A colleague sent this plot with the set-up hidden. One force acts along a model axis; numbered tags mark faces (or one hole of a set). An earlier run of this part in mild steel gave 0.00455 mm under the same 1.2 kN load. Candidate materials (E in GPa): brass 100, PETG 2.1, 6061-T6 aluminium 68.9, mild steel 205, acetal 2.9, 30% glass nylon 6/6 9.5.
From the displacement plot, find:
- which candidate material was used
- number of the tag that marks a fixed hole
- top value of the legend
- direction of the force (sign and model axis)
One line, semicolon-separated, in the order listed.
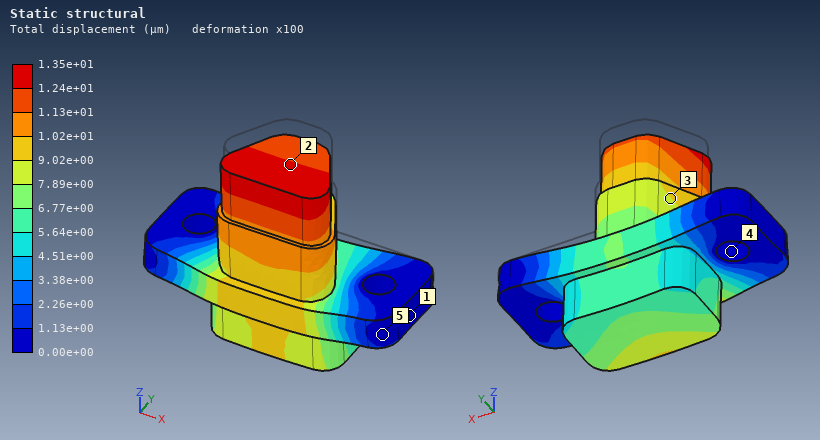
6061-T6 aluminium; 4; 1.35e+01 µm; -Z
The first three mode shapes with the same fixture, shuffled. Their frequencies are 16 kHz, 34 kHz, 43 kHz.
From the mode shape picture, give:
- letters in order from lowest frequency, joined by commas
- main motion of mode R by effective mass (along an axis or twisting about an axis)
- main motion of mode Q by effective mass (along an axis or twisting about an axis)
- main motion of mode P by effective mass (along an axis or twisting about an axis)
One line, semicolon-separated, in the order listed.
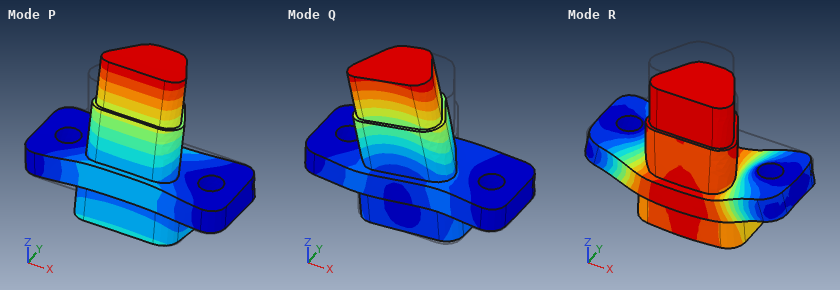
P, Q, R; along Z; along X; along Y
